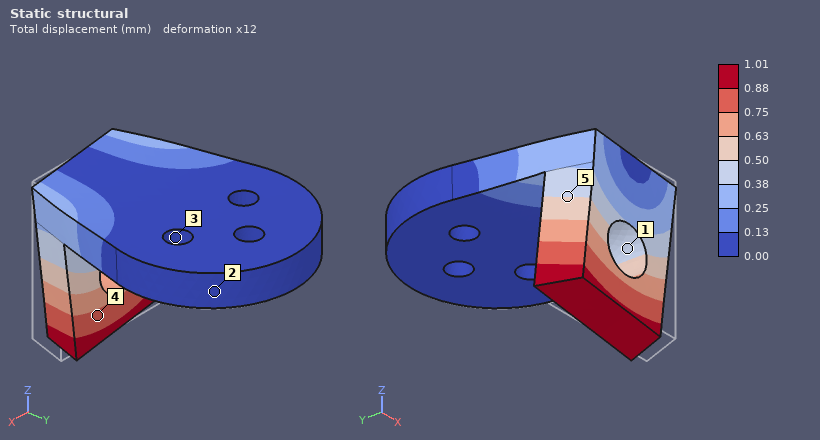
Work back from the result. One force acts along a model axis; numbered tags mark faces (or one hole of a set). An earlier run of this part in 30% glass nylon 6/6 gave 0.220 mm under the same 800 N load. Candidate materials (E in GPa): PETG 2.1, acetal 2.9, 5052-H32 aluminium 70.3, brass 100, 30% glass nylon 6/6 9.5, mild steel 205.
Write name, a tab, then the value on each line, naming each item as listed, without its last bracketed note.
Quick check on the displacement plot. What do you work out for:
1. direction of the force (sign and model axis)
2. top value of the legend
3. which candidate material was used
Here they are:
direction of the force	-X
top value of the legend	1.01 mm
which candidate material was used	PETG
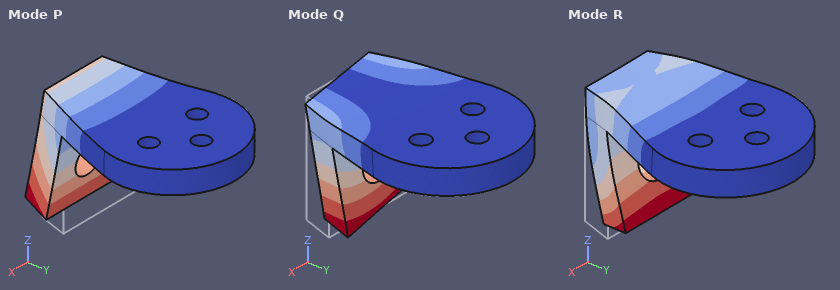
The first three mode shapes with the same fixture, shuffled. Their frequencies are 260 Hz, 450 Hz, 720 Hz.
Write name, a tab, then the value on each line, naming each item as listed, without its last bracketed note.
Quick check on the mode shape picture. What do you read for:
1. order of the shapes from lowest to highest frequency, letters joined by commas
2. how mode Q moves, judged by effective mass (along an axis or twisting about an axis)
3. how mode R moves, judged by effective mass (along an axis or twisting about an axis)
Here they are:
order of the shapes from lowest to highest frequency, letters joined by commas	P, Q, R
how mode Q moves, judged by effective mass	along X
how mode R moves, judged by effective mass	along Z
